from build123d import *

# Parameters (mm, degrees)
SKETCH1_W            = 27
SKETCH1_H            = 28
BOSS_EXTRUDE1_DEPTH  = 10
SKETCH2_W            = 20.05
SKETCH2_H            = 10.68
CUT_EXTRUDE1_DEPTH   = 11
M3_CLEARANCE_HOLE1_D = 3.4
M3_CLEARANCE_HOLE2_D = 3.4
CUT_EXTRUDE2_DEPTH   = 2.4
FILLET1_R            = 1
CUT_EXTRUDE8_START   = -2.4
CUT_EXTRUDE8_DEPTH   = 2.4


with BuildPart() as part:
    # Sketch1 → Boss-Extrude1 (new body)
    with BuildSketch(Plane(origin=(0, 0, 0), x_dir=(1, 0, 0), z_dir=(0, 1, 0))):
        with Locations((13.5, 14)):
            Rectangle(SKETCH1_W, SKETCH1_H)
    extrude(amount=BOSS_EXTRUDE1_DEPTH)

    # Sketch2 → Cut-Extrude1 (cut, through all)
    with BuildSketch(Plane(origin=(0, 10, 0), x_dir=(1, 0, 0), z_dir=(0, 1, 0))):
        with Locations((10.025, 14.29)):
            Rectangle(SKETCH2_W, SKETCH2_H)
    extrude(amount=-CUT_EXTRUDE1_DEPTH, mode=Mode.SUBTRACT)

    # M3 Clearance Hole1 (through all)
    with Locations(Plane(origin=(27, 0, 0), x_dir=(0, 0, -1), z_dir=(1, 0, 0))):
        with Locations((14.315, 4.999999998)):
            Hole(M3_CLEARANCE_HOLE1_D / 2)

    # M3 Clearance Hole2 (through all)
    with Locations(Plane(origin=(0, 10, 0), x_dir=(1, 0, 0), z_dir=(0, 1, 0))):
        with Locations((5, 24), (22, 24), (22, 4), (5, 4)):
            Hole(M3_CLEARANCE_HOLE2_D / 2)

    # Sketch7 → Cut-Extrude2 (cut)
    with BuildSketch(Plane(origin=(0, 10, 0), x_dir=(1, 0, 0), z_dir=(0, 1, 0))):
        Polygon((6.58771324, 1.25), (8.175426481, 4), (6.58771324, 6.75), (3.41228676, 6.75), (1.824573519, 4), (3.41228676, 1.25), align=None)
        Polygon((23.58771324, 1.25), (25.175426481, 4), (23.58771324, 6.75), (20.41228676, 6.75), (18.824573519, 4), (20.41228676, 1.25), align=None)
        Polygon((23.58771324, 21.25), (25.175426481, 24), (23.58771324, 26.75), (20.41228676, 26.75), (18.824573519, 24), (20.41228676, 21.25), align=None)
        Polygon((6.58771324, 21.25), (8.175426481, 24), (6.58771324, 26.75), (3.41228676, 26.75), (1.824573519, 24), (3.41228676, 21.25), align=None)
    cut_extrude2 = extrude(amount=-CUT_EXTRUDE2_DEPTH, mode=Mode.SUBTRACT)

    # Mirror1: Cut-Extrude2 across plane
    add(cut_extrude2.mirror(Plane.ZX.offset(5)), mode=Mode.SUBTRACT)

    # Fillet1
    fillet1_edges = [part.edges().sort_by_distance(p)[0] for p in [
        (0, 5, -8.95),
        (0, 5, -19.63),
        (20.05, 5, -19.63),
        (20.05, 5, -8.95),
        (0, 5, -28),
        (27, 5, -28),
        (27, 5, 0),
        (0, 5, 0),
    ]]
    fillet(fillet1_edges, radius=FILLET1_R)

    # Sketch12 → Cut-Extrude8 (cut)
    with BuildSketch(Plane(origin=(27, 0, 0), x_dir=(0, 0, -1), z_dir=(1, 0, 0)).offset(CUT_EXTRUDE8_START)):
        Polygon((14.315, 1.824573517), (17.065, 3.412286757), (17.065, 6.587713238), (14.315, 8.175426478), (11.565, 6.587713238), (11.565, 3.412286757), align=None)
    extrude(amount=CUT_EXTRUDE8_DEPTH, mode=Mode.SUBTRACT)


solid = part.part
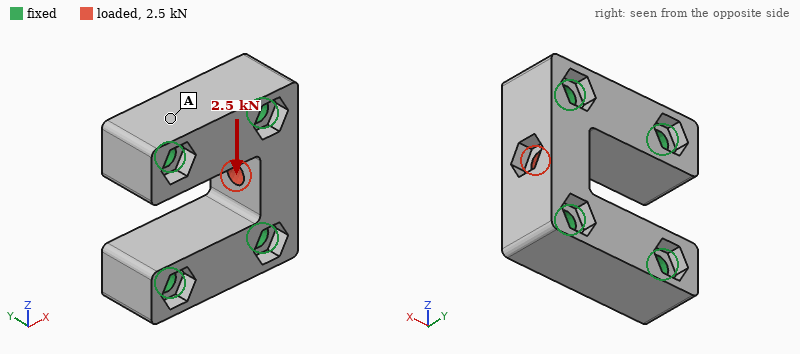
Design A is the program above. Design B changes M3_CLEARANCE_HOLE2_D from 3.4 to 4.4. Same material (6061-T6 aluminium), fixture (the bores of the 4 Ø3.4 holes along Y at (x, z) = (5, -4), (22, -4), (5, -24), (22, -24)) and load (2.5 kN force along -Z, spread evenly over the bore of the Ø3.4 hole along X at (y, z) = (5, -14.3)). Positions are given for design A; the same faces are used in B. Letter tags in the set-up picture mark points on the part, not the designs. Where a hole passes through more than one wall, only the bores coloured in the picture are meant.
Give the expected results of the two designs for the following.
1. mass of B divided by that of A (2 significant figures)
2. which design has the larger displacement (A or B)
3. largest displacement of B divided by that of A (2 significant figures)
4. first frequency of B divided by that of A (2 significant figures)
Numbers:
0.97
A
0.92
1.1
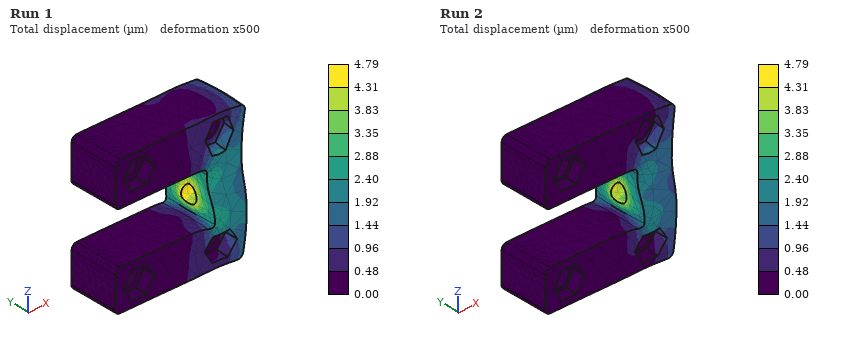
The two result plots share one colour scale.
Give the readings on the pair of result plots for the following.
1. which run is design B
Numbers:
Run 2
